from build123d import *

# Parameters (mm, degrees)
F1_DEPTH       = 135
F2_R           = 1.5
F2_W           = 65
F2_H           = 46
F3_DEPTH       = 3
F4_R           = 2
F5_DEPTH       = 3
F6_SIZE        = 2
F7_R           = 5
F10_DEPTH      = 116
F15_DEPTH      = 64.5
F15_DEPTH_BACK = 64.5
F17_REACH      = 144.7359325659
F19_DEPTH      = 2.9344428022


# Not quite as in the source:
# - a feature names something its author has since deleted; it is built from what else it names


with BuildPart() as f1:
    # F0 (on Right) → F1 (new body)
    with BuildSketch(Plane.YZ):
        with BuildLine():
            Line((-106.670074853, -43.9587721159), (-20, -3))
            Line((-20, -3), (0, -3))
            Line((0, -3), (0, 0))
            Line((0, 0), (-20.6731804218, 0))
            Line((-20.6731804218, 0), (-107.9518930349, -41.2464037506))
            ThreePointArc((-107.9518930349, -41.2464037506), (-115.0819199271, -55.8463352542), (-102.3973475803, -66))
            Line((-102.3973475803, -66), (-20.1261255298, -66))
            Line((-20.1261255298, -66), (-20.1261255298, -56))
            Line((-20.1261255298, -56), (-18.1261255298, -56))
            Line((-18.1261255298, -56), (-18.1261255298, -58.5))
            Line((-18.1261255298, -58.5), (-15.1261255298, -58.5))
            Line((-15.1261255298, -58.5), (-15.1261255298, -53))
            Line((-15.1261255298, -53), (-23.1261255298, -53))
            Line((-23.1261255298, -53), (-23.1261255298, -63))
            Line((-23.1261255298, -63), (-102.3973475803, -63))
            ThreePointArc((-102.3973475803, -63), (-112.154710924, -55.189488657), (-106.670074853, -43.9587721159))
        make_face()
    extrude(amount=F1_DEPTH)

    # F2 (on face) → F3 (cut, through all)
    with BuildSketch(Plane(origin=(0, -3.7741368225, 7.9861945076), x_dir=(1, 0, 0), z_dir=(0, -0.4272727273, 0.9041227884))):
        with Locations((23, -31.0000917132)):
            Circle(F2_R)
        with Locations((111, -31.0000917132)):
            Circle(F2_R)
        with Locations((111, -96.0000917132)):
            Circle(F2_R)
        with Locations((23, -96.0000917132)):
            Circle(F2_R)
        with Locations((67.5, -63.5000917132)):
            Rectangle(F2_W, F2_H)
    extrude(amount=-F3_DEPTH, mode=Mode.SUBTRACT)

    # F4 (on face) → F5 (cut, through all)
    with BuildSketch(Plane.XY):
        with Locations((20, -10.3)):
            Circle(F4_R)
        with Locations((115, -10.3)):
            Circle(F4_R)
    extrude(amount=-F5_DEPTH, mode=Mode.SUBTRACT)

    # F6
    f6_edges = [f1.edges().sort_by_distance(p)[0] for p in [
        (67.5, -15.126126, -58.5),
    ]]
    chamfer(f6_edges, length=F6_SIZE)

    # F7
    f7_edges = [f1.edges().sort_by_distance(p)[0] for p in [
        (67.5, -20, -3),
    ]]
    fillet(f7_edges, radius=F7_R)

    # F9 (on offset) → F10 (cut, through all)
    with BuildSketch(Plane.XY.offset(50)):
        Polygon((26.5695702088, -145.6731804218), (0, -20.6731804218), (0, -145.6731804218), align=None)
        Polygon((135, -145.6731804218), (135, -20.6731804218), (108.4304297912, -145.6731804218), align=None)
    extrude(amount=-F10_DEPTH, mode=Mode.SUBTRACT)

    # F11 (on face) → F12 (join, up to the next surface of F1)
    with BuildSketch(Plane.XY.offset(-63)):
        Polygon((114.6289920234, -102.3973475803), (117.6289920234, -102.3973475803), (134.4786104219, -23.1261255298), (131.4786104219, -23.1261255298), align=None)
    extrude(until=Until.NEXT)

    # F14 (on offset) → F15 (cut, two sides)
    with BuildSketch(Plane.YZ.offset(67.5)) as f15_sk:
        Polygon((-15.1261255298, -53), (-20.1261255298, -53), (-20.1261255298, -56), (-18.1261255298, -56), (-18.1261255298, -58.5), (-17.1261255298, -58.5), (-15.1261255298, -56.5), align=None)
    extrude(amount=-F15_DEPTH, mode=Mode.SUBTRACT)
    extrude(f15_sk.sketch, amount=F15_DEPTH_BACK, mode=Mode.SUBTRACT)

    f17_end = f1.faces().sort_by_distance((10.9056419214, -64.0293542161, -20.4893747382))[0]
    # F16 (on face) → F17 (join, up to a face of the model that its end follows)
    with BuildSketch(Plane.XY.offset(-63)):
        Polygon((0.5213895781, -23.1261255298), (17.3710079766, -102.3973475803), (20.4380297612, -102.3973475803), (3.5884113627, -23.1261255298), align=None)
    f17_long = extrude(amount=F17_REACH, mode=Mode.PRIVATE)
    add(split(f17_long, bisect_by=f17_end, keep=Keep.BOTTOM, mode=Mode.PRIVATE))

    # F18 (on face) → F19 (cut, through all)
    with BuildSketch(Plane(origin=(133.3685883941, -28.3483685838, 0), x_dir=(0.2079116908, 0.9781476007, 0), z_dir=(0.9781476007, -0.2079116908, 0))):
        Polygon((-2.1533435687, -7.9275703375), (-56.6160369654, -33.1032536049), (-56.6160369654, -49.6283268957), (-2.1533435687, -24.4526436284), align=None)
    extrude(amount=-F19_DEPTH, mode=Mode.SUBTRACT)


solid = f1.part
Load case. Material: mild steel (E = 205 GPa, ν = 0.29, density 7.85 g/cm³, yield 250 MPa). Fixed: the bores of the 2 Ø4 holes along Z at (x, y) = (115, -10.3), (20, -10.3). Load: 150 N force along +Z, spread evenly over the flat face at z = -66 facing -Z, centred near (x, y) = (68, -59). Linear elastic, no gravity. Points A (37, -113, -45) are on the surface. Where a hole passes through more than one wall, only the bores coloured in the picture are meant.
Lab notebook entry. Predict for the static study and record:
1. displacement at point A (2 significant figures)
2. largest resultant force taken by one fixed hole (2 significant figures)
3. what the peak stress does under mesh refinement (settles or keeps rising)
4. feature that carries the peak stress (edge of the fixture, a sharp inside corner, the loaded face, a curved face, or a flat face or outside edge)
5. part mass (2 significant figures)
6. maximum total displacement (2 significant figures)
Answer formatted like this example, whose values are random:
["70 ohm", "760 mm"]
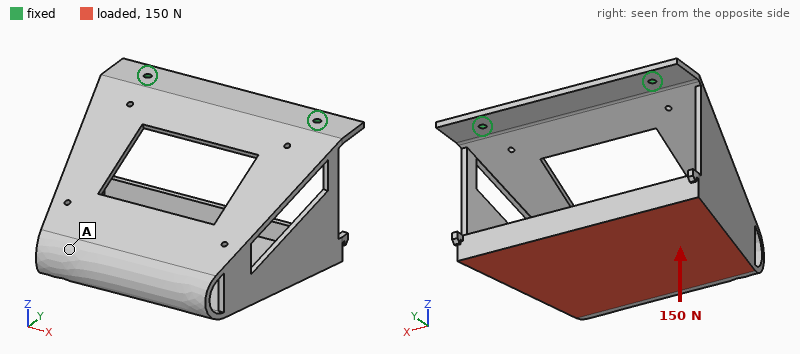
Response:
["0.41 mm", "78 N", "keeps rising", "edge of the fixture", "720 g", "0.44 mm"]
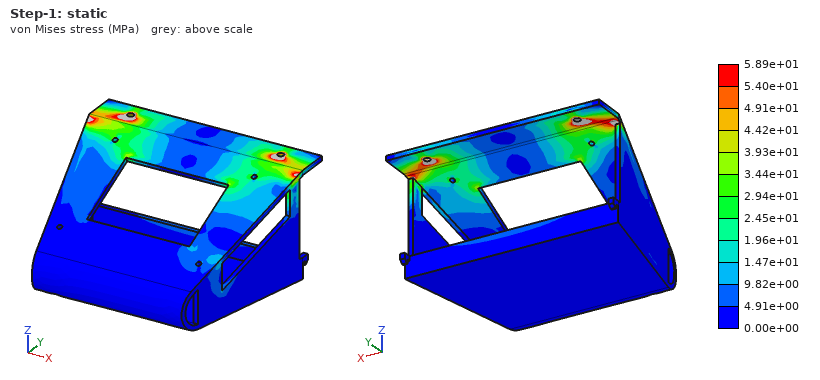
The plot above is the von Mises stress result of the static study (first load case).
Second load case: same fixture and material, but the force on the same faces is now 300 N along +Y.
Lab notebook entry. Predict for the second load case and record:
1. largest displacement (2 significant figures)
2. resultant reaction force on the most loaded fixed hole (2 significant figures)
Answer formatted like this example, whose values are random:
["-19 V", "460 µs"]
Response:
["1.4 mm", "150 N"]
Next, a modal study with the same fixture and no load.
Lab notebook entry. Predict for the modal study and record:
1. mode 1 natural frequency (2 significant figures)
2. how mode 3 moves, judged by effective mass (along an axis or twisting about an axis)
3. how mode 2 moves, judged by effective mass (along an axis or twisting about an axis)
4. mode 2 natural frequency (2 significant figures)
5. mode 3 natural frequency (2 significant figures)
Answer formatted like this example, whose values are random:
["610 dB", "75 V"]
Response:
["110 Hz", "along Z", "along X", "340 Hz", "1000 Hz"]
